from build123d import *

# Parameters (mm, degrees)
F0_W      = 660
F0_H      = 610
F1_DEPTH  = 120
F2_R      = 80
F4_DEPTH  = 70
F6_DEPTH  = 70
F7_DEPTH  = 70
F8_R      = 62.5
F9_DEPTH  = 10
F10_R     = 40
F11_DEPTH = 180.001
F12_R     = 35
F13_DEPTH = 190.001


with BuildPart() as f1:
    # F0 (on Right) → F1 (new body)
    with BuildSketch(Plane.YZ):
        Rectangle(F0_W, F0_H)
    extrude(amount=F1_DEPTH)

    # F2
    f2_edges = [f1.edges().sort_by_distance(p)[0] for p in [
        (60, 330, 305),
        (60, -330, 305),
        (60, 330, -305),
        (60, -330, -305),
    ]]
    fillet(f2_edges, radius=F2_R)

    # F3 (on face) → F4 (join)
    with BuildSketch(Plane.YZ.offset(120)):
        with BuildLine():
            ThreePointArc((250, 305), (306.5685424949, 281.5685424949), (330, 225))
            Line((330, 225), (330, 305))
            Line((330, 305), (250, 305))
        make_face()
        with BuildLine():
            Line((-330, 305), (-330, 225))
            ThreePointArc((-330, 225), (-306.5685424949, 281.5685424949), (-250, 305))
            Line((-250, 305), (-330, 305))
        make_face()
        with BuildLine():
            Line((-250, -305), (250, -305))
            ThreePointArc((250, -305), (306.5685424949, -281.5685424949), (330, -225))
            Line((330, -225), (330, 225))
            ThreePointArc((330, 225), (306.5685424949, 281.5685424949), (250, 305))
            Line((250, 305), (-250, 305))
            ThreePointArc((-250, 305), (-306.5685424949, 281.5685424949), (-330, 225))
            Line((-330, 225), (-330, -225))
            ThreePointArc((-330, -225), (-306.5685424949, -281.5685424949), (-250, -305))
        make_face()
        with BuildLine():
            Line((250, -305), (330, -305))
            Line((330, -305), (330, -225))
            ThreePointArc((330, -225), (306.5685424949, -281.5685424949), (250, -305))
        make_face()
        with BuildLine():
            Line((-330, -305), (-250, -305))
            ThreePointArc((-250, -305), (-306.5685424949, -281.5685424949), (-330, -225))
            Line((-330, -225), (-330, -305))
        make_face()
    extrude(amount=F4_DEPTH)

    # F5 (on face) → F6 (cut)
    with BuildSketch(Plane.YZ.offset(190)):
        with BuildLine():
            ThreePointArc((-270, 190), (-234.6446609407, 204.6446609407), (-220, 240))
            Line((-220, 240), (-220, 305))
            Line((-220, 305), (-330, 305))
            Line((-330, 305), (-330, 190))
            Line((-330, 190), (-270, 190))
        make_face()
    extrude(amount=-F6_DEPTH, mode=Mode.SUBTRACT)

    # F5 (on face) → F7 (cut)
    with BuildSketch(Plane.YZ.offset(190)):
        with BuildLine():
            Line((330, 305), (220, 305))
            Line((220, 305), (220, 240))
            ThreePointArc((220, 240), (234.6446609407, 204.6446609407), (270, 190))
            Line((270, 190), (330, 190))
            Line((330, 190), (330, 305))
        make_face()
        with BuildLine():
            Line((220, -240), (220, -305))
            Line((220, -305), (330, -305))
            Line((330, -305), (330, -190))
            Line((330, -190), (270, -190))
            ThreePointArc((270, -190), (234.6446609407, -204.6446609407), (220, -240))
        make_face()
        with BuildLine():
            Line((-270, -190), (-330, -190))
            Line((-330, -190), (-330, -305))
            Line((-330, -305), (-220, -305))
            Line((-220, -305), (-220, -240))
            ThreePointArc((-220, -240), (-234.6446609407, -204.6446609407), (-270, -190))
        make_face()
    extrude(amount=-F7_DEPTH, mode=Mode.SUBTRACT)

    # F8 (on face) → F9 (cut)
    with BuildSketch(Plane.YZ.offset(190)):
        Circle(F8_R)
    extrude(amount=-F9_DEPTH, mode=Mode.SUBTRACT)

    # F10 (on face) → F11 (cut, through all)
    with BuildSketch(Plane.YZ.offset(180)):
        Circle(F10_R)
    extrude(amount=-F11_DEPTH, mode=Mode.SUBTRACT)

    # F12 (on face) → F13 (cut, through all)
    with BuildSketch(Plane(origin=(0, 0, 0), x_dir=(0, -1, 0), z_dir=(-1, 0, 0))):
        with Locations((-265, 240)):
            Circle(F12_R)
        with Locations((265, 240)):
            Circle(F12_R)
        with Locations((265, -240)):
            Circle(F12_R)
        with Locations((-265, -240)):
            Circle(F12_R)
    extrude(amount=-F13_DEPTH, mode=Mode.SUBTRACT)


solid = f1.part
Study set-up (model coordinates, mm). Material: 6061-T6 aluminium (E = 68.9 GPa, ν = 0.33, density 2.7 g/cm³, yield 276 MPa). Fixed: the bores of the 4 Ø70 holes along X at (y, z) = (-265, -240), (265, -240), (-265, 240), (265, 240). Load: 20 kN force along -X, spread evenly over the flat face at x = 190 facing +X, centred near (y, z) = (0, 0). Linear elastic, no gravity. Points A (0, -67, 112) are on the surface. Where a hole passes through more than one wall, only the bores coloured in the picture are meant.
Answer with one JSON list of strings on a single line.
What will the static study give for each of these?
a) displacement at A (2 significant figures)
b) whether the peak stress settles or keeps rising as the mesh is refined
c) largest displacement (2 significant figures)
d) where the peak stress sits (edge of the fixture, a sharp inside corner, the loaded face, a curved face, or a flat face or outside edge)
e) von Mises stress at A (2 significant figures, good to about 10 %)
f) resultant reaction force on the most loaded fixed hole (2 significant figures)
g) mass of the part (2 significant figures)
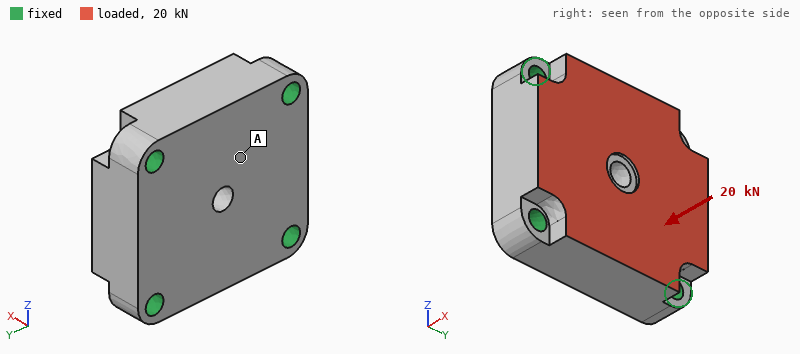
["1.4 µm", "keeps rising", "1.6 µm", "edge of the fixture", "0.13 MPa", "5.4 kN", "190 kg"]
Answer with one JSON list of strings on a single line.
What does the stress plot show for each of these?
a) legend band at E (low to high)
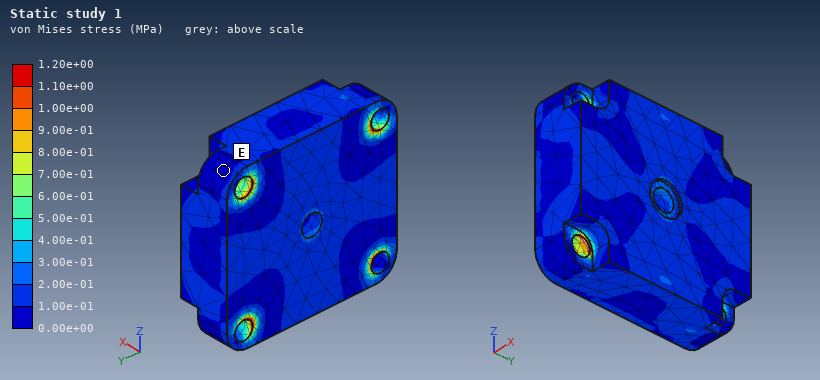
["0.00e+00 to 1.00e-01 MPa"]
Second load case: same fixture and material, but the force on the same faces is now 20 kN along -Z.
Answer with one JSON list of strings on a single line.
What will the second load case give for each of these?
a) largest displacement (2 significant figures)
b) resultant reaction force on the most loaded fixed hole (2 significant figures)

["1.5 µm", "5.8 kN"]
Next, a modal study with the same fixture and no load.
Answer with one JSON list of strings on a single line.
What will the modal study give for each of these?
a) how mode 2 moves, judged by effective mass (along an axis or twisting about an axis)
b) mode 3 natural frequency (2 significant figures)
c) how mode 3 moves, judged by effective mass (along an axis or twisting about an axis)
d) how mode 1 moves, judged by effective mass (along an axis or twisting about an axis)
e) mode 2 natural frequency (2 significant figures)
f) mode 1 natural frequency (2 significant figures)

["twisting about Y", "2300 Hz", "along Z", "along X", "2100 Hz", "1500 Hz"]
